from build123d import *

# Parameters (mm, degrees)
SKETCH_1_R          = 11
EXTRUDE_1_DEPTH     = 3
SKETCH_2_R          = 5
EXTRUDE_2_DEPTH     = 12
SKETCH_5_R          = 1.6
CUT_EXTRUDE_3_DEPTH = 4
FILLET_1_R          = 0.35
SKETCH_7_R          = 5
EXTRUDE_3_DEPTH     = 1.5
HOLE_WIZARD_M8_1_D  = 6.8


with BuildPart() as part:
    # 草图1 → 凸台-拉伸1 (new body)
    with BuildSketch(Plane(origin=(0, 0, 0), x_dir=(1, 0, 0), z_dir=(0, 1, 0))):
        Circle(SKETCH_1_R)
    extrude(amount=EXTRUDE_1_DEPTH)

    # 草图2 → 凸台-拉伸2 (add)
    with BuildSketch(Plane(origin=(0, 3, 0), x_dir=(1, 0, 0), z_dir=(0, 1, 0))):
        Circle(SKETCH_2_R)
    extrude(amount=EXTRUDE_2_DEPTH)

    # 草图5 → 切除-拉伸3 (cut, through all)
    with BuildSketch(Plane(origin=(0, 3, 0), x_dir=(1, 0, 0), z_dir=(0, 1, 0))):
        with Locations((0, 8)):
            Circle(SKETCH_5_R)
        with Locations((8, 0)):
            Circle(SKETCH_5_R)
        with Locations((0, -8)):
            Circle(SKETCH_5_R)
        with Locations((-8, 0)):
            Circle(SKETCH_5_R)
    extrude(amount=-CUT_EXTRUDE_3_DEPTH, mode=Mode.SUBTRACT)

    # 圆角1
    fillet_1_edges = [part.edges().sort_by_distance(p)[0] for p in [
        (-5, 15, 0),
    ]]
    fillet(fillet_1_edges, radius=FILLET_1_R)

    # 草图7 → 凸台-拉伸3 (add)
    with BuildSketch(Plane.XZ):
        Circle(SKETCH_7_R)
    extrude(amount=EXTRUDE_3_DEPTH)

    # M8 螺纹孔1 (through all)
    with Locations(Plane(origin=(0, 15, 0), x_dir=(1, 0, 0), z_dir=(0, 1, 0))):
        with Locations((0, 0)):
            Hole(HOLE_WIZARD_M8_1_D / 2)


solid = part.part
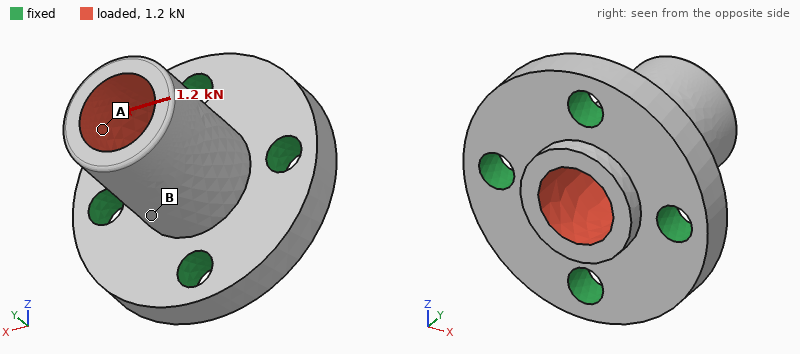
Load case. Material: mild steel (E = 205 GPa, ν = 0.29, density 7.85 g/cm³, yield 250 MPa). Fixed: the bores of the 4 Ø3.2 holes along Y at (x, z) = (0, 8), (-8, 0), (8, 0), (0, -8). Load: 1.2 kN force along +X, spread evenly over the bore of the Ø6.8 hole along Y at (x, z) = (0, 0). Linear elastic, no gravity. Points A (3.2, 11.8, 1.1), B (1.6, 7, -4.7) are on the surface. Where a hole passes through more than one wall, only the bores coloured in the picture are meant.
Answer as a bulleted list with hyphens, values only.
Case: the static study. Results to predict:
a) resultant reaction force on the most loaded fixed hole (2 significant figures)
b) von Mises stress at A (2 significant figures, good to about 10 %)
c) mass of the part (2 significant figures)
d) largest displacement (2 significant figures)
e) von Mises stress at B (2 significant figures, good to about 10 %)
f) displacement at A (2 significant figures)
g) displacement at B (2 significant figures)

- 590 N
- 15 MPa
- 12 g
- 9.0 µm
- 35 MPa
- 6.9 µm
- 3.3 µm
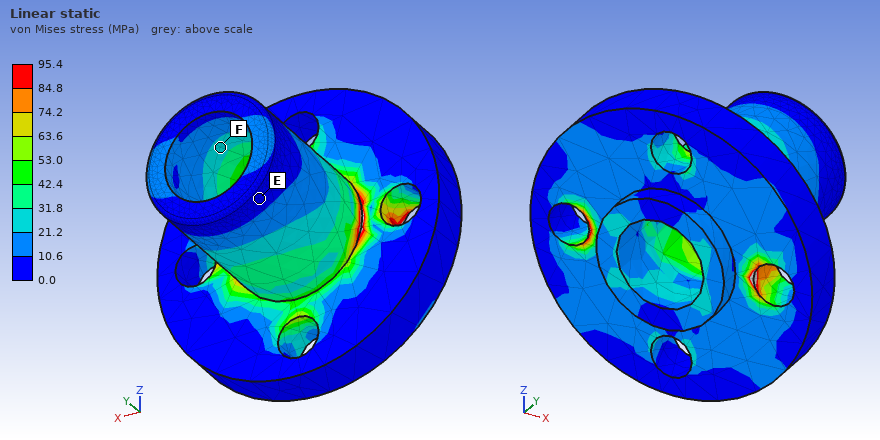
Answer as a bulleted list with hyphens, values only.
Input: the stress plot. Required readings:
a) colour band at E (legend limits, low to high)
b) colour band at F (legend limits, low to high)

- 0.0 to 10.6 MPa
- 21.2 to 31.8 MPa
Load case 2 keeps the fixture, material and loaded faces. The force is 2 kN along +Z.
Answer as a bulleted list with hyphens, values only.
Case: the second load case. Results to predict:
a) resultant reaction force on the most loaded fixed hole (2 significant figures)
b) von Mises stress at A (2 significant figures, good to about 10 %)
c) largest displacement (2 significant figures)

- 980 N
- 38 MPa
- 15 µm
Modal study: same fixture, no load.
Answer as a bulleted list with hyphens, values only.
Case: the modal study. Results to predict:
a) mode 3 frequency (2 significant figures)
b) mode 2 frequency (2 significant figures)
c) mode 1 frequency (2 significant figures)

- 60 kHz
- 29 kHz
- 29 kHz
